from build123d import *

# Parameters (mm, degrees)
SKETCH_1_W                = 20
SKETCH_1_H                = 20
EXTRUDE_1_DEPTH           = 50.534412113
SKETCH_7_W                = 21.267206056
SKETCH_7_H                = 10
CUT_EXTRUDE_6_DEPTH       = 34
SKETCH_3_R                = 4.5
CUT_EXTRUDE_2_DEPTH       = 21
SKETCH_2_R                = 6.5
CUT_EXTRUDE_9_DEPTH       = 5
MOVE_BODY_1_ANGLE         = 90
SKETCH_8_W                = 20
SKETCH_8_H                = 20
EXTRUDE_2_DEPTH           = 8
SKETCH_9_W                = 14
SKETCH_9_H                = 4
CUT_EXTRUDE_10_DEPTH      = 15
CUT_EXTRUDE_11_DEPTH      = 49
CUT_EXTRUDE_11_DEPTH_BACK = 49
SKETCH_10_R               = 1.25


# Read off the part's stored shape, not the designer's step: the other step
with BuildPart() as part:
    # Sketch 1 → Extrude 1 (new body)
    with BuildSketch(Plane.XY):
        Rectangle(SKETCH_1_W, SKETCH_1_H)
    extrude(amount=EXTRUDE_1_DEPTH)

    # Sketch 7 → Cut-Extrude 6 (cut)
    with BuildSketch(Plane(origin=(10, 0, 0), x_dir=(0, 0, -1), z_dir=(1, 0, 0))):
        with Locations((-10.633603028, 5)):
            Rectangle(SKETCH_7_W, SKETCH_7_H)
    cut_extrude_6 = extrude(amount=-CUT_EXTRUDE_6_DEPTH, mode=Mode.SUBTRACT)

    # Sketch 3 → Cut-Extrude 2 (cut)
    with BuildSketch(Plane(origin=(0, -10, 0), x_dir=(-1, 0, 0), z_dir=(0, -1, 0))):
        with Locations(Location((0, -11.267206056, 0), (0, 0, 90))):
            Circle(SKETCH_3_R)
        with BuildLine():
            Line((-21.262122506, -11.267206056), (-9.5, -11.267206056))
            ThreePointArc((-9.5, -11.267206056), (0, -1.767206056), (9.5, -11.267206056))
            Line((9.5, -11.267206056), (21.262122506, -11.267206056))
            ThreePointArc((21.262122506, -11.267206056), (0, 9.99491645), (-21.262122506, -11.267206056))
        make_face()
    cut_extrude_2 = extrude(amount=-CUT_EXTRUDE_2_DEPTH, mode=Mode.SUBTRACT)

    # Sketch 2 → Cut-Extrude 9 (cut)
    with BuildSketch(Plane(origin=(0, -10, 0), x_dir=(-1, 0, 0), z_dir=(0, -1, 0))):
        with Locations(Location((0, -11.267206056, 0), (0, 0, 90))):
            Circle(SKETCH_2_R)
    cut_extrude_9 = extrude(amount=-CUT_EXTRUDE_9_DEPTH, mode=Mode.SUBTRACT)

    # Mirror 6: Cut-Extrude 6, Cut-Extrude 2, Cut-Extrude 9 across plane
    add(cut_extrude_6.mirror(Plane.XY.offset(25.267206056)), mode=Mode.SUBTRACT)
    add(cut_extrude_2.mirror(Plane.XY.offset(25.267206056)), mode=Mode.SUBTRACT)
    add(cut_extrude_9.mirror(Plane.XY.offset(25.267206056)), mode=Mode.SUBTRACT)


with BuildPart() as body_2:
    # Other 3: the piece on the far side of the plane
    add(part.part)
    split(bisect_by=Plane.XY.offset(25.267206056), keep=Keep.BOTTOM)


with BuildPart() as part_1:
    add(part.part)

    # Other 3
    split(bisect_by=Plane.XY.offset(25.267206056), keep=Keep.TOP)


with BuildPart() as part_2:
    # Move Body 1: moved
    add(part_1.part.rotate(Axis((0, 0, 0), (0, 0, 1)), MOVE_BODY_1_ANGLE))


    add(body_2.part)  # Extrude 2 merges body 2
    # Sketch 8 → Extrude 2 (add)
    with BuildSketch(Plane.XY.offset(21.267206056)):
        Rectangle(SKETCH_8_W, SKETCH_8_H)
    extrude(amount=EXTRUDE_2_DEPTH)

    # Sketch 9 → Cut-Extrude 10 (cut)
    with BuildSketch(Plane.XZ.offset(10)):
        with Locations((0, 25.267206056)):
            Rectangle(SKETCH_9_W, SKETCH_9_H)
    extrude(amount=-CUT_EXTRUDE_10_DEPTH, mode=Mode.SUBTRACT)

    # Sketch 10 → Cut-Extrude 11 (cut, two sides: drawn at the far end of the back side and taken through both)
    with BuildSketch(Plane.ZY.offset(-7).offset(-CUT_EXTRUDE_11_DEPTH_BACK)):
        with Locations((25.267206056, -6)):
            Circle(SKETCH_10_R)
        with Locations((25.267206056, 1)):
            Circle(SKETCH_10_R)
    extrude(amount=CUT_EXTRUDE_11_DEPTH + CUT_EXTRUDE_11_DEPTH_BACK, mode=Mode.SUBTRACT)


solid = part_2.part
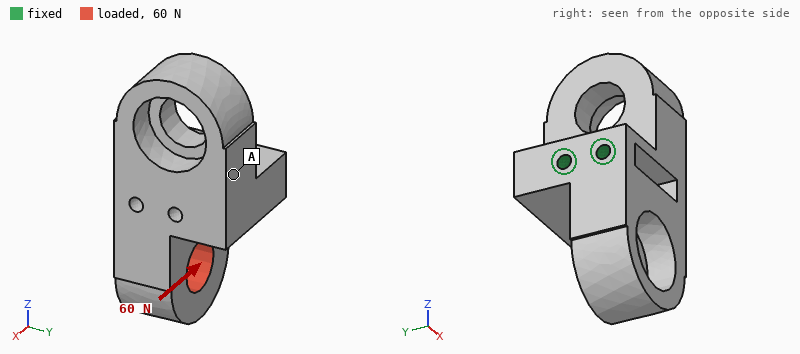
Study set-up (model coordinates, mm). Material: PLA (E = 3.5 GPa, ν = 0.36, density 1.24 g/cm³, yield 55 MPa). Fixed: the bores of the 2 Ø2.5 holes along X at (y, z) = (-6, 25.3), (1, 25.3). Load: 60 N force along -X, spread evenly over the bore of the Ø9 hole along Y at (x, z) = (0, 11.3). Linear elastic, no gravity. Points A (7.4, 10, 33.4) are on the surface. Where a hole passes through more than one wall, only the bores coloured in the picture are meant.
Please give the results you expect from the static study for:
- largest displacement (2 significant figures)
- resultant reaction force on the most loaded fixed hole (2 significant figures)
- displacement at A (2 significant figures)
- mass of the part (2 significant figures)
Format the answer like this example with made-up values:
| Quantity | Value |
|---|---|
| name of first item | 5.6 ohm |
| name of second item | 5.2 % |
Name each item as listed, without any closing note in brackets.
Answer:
| Quantity | Value |
|---|---|
| largest displacement | 0.26 mm |
| resultant reaction force on the most loaded fixed hole | 32 N |
| displacement at A | 0.14 mm |
| mass of the part | 8.9 g |
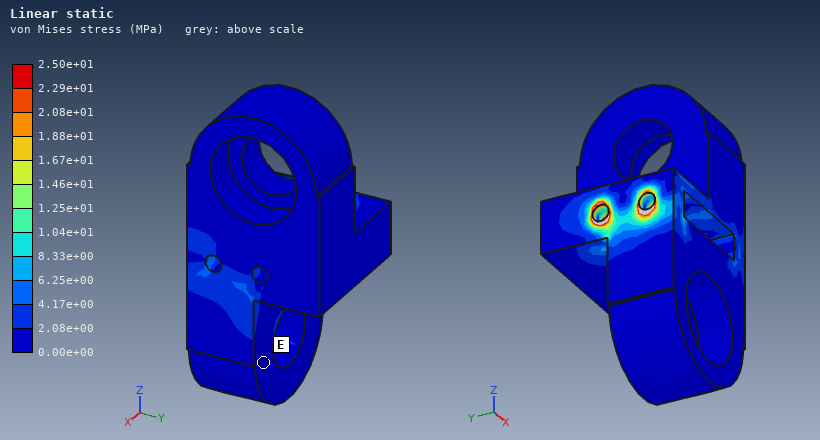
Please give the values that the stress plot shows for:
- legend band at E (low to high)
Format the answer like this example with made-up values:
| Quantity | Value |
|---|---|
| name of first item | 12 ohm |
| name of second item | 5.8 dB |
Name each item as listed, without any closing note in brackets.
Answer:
| Quantity | Value |
|---|---|
| legend band at E | 0.00e+00 to 2.08e+00 MPa |
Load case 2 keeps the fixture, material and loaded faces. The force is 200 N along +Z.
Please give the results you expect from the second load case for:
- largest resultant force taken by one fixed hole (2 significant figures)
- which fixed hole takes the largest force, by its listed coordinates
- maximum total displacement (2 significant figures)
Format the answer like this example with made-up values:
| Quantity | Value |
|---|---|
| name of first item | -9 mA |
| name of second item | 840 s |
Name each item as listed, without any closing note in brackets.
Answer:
| Quantity | Value |
|---|---|
| largest resultant force taken by one fixed hole | 110 N |
| which fixed hole takes the largest force, by its listed coordinates | (-6, 25.3) |
| maximum total displacement | 0.58 mm |
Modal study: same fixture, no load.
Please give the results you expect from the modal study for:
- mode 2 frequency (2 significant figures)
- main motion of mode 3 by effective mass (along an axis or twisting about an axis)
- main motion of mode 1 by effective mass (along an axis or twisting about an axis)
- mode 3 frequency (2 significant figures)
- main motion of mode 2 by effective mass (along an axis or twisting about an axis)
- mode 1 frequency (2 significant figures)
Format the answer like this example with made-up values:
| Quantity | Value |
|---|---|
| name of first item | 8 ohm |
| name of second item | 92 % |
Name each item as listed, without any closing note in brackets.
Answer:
| Quantity | Value |
|---|---|
| mode 2 frequency | 1900 Hz |
| main motion of mode 3 by effective mass | along Y |
| main motion of mode 1 by effective mass | along Z |
| mode 3 frequency | 2500 Hz |
| main motion of mode 2 by effective mass | along Y |
| mode 1 frequency | 990 Hz |
